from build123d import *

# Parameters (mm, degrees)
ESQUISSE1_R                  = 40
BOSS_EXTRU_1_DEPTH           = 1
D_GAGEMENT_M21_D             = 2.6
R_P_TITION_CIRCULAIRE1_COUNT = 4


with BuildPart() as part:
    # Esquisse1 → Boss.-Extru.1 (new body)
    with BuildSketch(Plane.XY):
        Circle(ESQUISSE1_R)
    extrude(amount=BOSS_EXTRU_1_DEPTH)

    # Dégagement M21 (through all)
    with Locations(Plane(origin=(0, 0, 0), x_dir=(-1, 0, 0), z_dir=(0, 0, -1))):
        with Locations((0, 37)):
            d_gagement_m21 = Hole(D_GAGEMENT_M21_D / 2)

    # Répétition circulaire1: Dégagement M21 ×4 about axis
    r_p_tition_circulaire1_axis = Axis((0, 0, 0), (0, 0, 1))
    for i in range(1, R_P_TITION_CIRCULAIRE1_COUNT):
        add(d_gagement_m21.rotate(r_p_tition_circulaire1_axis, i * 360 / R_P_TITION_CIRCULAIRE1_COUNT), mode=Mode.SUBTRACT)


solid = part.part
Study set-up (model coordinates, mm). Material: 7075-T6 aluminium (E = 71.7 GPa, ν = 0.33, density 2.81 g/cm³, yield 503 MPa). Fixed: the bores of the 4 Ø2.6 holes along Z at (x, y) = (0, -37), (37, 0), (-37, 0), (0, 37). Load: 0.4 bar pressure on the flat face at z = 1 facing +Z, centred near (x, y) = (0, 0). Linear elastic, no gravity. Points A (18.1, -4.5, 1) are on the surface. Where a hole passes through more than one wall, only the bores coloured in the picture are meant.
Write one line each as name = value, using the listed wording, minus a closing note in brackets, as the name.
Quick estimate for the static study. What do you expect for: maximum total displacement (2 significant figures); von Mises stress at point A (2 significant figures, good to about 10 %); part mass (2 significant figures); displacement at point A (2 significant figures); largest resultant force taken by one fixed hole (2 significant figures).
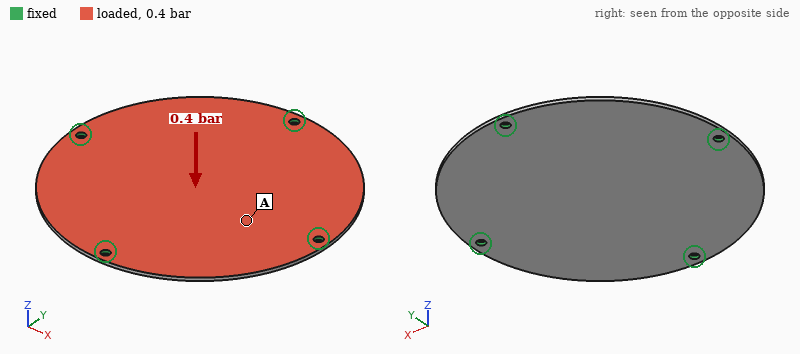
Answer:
maximum total displacement = 0.31 mm
von Mises stress at point A = 22 MPa
part mass = 14 g
displacement at point A = 0.21 mm
largest resultant force taken by one fixed hole = 50 N
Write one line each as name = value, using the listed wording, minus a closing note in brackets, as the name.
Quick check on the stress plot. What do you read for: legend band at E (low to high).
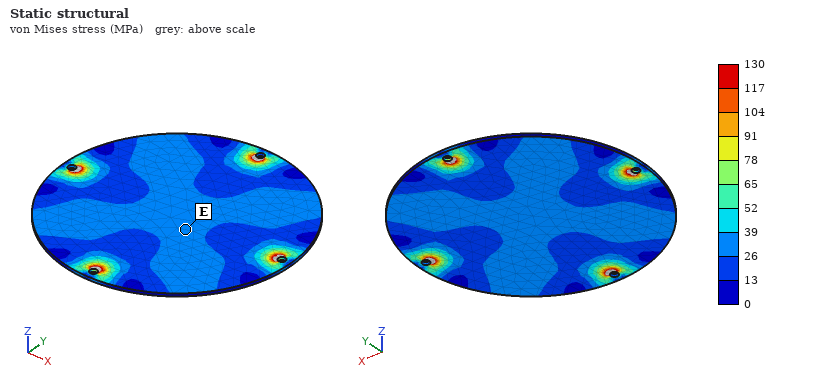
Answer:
legend band at E = 26 to 39 MPa
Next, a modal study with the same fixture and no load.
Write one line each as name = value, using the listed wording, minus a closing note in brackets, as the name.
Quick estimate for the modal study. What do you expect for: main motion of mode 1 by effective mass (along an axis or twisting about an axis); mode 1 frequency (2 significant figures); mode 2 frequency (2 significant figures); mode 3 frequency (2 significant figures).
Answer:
main motion of mode 1 by effective mass = along Z
mode 1 frequency = 1300 Hz
mode 2 frequency = 1600 Hz
mode 3 frequency = 1700 Hz
